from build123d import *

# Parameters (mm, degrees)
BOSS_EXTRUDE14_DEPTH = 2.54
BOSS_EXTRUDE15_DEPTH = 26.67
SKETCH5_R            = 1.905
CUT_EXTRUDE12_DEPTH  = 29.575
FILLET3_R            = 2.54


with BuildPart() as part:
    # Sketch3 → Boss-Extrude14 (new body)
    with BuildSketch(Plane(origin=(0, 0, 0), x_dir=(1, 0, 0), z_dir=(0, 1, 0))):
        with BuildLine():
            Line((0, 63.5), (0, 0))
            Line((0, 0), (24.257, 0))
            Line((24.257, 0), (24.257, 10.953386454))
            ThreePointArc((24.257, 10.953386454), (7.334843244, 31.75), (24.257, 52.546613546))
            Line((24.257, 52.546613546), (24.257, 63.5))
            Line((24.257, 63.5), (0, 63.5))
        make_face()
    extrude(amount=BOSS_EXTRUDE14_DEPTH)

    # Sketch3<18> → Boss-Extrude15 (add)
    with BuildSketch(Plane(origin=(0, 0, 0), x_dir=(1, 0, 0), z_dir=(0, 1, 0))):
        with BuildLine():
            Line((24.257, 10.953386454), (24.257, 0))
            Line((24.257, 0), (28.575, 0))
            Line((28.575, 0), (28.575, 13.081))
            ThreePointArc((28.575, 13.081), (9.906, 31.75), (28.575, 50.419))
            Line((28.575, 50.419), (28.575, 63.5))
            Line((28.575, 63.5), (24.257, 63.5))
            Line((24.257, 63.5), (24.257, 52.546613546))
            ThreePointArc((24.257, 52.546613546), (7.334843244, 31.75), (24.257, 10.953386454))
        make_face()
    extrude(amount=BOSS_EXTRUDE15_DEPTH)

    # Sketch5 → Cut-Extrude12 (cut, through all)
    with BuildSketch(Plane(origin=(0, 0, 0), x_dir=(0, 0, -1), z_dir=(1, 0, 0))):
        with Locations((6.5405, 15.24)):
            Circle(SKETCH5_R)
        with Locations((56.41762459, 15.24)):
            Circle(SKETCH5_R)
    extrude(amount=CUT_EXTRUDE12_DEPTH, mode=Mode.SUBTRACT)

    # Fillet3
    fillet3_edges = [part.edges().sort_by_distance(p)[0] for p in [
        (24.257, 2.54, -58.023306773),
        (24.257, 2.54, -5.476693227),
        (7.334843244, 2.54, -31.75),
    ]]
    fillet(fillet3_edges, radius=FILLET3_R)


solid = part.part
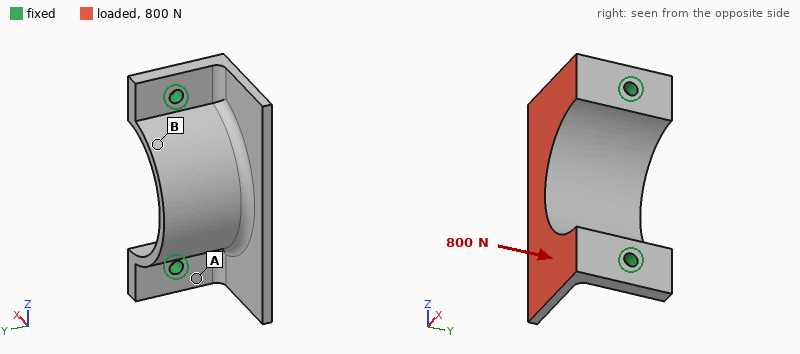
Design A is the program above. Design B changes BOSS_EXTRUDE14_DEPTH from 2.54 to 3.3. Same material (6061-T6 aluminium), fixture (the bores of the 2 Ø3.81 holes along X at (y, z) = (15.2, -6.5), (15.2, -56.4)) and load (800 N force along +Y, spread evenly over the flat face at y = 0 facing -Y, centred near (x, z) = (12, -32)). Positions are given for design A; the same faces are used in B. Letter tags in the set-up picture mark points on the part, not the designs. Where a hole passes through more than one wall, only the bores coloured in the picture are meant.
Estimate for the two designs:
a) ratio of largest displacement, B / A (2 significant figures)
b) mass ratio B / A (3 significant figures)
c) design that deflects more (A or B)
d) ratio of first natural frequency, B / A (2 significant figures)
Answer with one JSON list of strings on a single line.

["0.76", "1.08", "A", "0.95"]
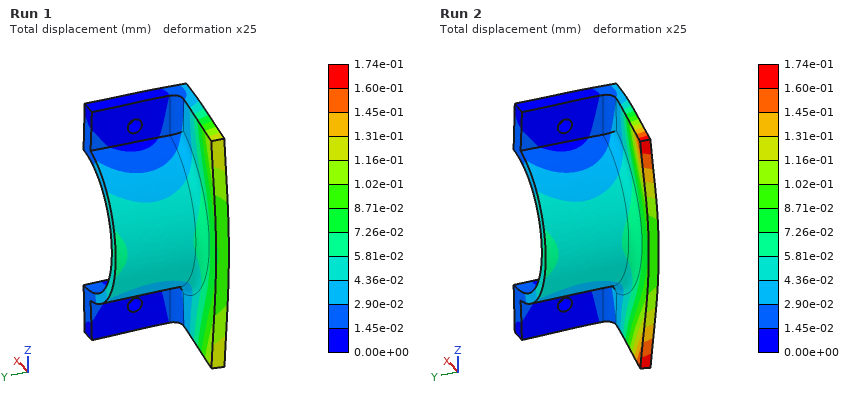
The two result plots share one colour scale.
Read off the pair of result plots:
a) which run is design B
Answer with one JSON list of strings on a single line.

["Run 1"]
